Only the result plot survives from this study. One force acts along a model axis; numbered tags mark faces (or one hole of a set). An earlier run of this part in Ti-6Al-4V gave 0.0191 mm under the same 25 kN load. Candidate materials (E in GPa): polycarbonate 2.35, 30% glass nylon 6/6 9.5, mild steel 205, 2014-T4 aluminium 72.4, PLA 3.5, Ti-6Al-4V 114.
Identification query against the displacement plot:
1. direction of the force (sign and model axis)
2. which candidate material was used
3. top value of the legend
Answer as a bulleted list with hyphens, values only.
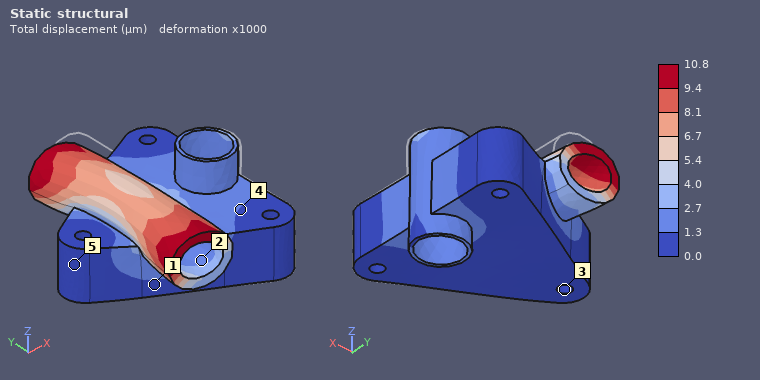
- -X
- mild steel
- 10.8 µm
